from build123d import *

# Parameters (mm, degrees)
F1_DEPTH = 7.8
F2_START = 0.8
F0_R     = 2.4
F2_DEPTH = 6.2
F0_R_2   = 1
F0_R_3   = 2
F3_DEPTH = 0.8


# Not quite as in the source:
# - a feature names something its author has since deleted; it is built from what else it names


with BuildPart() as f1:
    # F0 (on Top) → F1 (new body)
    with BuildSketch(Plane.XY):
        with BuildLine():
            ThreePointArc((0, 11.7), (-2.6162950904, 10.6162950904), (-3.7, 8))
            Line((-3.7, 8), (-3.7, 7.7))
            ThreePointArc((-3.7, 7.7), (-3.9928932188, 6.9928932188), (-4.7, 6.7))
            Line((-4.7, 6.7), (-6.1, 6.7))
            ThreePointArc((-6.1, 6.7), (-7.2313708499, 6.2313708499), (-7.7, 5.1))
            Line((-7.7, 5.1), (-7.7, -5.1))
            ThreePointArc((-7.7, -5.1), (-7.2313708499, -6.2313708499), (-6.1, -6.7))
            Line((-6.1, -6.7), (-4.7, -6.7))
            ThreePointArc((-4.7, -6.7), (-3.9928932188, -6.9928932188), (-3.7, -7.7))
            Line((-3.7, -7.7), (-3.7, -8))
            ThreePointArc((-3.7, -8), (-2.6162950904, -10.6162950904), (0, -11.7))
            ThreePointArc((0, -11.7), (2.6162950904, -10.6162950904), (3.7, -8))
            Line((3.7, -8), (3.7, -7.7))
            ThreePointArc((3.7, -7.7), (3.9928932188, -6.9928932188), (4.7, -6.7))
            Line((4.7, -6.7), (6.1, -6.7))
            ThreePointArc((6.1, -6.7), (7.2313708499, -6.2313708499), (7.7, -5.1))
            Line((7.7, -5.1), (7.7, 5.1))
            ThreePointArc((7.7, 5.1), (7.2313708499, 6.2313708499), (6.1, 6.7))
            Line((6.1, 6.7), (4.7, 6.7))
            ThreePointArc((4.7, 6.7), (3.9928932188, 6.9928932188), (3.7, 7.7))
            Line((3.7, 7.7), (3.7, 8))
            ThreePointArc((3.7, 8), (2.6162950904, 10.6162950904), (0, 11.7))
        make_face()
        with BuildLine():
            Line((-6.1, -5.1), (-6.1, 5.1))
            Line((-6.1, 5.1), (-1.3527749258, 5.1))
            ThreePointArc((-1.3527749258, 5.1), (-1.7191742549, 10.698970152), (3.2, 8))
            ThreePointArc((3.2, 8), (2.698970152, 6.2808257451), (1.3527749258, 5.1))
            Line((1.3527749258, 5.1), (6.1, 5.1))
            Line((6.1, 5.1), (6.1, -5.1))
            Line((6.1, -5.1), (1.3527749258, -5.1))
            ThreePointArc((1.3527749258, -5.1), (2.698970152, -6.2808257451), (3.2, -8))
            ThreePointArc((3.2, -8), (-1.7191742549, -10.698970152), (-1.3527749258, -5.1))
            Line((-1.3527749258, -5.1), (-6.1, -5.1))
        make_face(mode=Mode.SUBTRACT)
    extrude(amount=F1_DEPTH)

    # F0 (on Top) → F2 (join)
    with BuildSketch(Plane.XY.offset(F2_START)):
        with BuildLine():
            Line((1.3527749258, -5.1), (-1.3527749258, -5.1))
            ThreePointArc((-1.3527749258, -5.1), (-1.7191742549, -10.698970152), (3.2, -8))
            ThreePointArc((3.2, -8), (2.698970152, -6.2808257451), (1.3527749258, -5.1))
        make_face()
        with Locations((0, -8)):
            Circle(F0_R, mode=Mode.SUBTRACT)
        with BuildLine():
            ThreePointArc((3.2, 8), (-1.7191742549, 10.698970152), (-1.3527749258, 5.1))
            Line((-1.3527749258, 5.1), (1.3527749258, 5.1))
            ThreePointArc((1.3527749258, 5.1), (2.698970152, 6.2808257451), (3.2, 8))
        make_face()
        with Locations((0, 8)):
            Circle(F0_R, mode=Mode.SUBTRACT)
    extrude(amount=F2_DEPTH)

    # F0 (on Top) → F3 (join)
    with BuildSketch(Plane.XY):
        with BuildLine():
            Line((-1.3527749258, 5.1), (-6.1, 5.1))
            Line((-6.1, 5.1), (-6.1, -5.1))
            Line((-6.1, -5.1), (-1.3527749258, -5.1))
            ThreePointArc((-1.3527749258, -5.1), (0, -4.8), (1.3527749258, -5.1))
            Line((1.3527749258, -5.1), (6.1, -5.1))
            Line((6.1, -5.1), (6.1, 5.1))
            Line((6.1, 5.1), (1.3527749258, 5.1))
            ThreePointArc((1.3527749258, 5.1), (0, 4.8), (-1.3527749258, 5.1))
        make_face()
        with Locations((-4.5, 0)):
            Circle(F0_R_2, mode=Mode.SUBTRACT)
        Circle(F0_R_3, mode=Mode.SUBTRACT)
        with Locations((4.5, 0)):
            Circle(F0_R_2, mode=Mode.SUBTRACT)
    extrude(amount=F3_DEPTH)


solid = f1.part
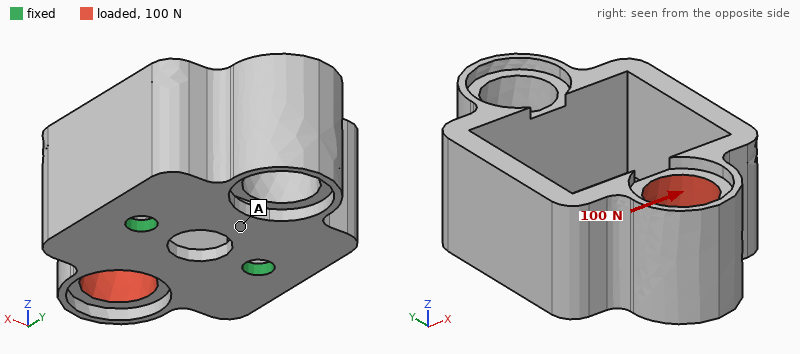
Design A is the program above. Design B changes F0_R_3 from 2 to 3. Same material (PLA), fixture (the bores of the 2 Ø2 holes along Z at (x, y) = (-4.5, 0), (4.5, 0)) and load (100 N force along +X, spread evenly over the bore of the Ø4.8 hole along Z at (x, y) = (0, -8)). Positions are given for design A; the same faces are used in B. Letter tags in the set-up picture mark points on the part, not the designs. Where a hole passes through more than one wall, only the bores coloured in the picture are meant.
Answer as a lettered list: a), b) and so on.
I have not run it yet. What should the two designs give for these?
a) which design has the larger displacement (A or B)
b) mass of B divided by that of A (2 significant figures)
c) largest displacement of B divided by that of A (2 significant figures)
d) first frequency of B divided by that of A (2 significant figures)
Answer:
a) B
b) 0.99
c) 1.1
d) 0.96
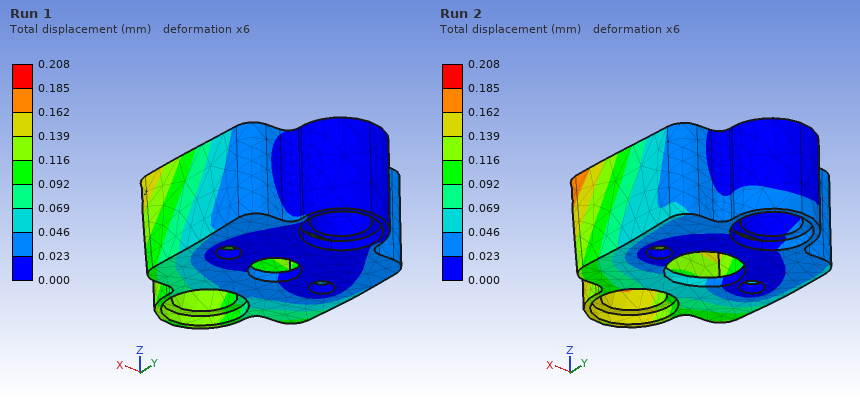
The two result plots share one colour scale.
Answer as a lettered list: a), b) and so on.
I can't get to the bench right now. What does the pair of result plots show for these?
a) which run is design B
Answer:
a) Run 2
